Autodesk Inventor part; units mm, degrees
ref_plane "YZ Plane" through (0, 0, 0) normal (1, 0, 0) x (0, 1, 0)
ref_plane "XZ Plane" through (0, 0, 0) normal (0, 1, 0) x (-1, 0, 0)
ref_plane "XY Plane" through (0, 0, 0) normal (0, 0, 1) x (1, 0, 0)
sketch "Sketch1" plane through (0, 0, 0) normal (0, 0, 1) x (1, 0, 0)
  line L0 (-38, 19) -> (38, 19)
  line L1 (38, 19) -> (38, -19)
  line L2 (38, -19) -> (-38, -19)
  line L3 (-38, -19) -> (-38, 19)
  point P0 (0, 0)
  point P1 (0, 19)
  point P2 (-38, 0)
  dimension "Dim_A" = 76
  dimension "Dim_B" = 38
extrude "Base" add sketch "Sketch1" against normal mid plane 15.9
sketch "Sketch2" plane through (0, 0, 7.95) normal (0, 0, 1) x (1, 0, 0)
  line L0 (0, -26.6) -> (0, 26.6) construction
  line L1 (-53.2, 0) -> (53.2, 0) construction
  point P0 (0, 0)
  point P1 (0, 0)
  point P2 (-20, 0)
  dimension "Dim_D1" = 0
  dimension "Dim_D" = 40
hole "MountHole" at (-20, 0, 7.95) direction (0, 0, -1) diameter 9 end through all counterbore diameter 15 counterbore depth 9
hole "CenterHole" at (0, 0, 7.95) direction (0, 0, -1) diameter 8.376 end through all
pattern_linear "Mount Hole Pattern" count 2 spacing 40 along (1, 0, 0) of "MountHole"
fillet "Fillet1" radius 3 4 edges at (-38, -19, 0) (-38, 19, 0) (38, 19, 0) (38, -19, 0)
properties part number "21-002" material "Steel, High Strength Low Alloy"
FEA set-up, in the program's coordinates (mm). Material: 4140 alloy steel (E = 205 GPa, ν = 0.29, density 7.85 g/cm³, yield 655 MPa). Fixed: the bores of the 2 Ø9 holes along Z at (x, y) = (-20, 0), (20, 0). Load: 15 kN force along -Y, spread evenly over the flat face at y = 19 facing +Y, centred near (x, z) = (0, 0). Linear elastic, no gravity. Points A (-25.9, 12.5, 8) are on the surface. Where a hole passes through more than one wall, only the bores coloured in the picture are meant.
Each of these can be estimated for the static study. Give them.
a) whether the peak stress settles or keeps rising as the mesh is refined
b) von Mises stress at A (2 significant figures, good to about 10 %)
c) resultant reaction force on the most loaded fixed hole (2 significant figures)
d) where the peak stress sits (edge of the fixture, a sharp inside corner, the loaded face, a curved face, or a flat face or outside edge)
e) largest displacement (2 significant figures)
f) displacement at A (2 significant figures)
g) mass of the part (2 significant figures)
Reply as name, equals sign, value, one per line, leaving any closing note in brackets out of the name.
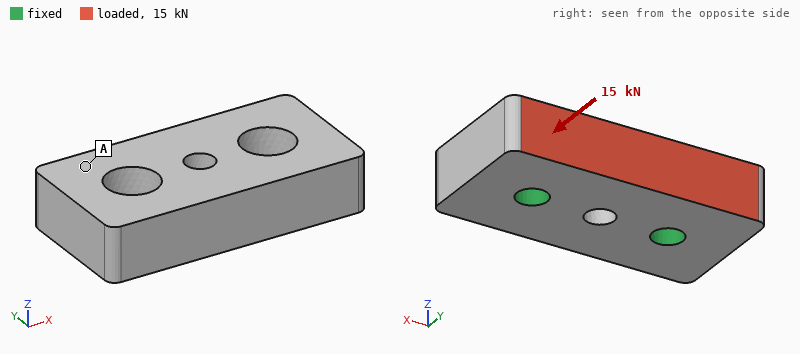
whether the peak stress settles or keeps rising as the mesh is refined = keeps rising
von Mises stress at A = 18 MPa
resultant reaction force on the most loaded fixed hole = 7.5 kN
where the peak stress sits = edge of the fixture
largest displacement = 12 µm
displacement at A = 9.4 µm
mass of the part = 320 g
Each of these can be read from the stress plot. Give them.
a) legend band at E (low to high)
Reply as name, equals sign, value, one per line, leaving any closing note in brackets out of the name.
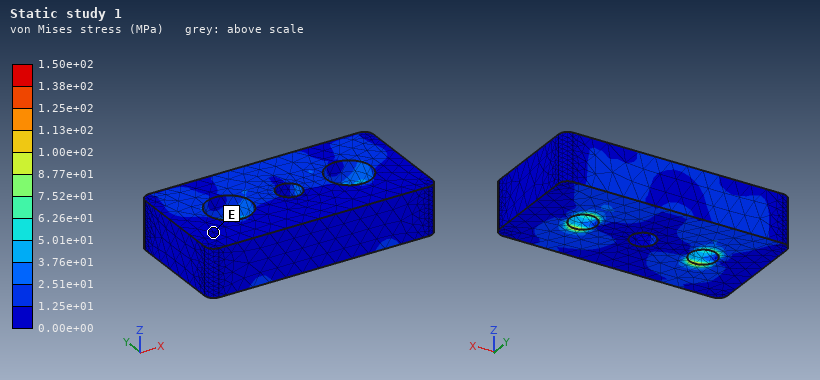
legend band at E = 0.00e+00 to 1.25e+01 MPa
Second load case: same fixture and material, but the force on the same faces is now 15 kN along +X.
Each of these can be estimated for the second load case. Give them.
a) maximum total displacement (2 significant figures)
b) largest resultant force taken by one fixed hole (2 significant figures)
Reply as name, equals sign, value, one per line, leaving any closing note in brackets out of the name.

maximum total displacement = 11 µm
largest resultant force taken by one fixed hole = 9.5 kN
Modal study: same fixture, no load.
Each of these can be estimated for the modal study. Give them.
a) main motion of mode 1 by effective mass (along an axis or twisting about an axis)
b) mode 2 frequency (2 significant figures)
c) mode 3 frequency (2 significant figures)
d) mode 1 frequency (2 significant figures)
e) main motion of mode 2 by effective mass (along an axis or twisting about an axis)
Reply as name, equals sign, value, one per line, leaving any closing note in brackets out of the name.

main motion of mode 1 by effective mass = along Y
mode 2 frequency = 14 kHz
mode 3 frequency = 16 kHz
mode 1 frequency = 9100 Hz
main motion of mode 2 by effective mass = twisting about Z
